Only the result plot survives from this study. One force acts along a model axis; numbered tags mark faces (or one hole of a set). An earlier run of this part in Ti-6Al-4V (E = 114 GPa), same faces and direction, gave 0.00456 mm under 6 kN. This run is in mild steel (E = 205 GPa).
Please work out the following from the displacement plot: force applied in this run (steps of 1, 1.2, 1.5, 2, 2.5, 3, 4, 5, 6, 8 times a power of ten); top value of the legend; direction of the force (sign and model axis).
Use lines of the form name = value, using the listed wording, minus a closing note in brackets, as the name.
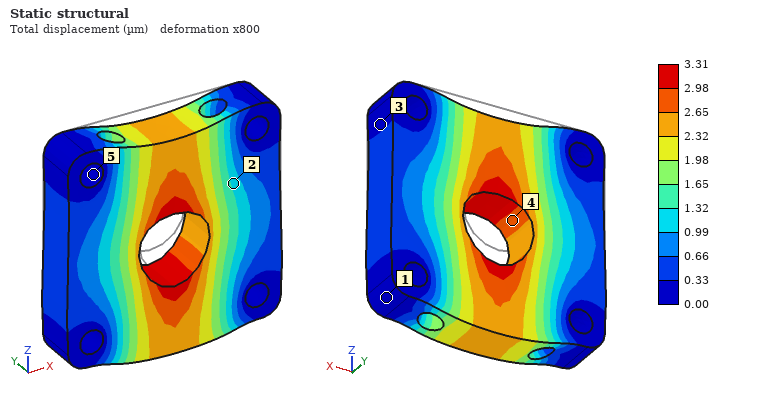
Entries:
force applied in this run = 8 kN
top value of the legend = 3.31 µm
direction of the force = -Z
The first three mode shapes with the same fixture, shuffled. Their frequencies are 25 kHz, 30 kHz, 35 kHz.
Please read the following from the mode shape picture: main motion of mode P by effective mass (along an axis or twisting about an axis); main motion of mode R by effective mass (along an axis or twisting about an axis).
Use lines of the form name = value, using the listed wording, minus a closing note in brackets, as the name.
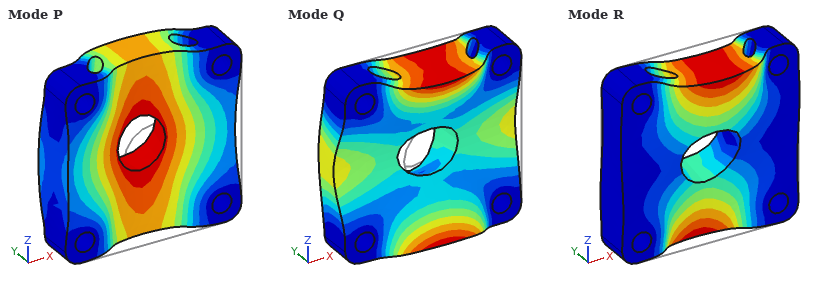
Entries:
main motion of mode P by effective mass = along Y
main motion of mode R by effective mass = twisting about X
